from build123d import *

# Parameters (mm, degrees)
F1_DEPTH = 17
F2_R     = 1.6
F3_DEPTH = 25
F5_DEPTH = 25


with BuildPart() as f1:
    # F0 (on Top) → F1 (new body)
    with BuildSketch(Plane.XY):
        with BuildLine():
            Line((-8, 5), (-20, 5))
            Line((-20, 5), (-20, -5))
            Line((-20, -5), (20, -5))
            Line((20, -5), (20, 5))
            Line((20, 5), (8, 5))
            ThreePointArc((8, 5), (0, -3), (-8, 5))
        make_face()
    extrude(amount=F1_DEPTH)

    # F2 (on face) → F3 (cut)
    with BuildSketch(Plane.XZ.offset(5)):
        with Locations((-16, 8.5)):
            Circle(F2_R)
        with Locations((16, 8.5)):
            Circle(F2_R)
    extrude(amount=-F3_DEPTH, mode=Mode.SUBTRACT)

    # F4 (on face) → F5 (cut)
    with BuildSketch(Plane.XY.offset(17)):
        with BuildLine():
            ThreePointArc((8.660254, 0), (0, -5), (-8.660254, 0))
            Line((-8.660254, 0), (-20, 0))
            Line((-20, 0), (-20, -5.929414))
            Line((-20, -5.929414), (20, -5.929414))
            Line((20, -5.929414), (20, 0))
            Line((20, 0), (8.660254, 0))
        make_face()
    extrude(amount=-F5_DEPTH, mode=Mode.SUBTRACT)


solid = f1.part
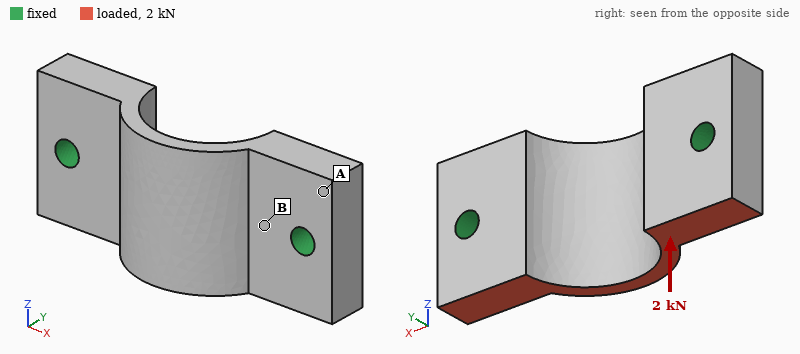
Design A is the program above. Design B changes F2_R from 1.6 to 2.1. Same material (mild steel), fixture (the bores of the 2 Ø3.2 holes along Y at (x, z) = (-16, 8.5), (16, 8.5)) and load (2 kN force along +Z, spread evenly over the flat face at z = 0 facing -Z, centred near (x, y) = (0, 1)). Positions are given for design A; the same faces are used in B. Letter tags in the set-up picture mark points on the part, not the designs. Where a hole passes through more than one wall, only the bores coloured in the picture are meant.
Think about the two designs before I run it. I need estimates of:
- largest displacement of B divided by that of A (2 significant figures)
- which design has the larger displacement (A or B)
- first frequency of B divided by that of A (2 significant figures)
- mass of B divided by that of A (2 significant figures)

0.75
A
1.2
0.98
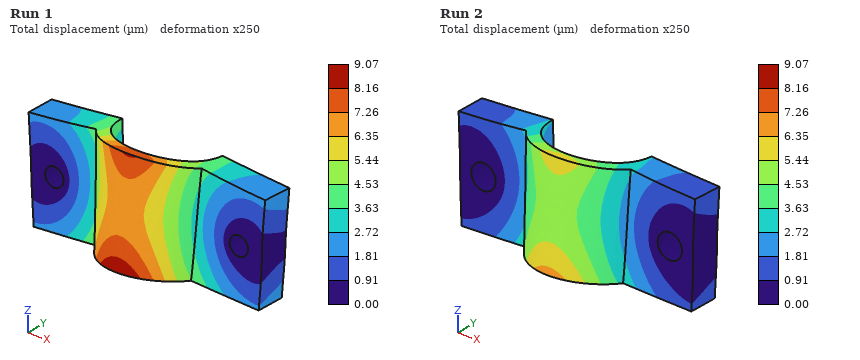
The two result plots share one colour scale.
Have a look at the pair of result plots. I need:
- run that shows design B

Run 2
